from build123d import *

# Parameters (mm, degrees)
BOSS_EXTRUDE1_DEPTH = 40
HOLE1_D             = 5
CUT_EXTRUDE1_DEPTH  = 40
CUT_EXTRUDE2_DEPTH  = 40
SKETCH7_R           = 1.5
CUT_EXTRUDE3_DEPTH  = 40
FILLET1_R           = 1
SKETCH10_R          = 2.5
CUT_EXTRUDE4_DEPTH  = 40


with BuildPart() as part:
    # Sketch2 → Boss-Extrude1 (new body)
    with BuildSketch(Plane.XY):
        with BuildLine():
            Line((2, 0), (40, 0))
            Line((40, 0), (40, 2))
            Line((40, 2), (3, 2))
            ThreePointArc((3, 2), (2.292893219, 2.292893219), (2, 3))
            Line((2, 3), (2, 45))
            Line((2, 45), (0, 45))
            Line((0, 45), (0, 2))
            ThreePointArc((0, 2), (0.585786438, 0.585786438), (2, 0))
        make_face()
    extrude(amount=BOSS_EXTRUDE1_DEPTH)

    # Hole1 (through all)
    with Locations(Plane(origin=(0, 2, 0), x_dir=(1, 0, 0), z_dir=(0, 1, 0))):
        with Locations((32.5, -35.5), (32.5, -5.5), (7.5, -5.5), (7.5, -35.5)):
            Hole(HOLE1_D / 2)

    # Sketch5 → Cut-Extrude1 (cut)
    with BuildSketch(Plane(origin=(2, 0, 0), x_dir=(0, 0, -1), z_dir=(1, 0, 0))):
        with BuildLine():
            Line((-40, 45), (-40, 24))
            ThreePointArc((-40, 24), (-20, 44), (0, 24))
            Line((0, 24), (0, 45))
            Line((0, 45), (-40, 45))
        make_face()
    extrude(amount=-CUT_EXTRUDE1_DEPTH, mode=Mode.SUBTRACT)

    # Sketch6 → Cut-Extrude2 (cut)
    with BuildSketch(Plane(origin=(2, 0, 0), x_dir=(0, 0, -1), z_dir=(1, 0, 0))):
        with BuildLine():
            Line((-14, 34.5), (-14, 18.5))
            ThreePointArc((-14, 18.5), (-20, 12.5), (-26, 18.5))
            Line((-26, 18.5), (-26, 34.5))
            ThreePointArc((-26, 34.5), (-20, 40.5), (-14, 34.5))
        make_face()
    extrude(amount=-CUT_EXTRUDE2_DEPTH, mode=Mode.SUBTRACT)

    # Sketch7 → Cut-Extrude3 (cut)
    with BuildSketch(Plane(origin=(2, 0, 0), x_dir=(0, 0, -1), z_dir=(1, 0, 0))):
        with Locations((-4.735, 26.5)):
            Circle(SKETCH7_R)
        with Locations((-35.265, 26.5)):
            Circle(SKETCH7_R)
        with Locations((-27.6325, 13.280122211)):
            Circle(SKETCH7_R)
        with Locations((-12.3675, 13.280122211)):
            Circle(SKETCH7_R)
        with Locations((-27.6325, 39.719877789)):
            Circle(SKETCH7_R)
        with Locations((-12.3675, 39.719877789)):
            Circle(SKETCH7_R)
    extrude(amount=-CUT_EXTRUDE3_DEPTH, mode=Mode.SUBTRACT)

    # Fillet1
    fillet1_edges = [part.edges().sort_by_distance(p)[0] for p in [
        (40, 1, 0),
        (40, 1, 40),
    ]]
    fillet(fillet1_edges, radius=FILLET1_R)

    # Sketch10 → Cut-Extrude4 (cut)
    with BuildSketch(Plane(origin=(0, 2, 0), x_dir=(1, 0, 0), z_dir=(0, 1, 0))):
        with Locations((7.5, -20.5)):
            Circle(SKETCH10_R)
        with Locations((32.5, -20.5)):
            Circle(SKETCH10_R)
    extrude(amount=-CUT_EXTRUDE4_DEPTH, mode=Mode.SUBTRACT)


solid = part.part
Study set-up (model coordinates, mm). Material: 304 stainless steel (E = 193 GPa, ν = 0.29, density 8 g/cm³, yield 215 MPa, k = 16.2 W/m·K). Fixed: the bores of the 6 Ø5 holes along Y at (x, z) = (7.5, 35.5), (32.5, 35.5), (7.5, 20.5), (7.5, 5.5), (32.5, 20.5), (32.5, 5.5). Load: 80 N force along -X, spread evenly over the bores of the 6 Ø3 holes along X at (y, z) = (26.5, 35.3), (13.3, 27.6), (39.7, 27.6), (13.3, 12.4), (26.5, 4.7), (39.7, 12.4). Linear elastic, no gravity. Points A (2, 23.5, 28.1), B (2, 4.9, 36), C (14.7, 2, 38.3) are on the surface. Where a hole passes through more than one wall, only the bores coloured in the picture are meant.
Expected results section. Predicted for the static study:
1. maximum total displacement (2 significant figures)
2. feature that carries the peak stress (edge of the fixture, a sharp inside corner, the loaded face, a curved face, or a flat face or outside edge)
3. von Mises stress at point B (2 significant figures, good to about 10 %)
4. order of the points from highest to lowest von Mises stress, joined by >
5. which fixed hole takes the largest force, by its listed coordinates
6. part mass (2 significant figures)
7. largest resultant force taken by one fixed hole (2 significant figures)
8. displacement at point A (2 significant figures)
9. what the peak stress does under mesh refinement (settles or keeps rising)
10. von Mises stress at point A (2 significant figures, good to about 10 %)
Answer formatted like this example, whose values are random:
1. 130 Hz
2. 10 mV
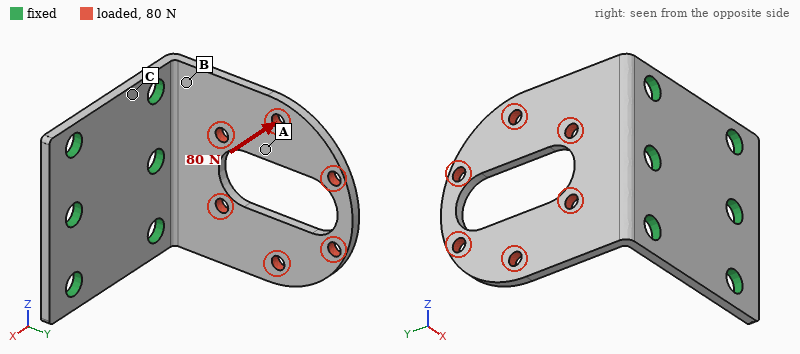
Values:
1. 0.28 mm
2. edge of the fixture
3. 61 MPa
4. B > A > C
5. (7.5, 20.5)
6. 42 g
7. 41 N
8. 0.11 mm
9. keeps rising
10. 33 MPa
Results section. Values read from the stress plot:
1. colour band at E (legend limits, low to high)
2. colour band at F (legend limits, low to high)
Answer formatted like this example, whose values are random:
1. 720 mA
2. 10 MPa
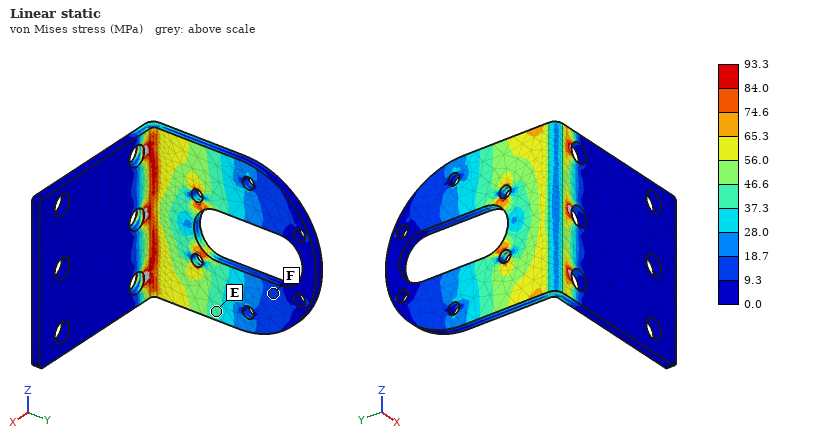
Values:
1. 37.3 to 46.6 MPa
2. 9.3 to 18.7 MPa
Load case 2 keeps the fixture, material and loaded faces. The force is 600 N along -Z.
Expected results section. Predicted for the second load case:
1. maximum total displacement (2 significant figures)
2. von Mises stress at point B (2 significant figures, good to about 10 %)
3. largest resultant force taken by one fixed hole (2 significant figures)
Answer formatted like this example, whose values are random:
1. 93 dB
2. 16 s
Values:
1. 51 µm
2. 68 MPa
3. 530 N
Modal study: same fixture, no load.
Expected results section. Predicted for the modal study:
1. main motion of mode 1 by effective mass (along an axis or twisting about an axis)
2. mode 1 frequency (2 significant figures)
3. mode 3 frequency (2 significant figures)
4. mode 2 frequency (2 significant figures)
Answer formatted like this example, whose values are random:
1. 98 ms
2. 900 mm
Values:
1. along X
2. 1000 Hz
3. 4900 Hz
4. 2300 Hz
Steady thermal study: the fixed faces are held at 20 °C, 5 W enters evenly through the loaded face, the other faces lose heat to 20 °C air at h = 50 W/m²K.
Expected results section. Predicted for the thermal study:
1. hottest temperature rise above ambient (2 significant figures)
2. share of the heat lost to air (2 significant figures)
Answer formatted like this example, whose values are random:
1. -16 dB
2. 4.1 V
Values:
1. 54 K
2. 73 %
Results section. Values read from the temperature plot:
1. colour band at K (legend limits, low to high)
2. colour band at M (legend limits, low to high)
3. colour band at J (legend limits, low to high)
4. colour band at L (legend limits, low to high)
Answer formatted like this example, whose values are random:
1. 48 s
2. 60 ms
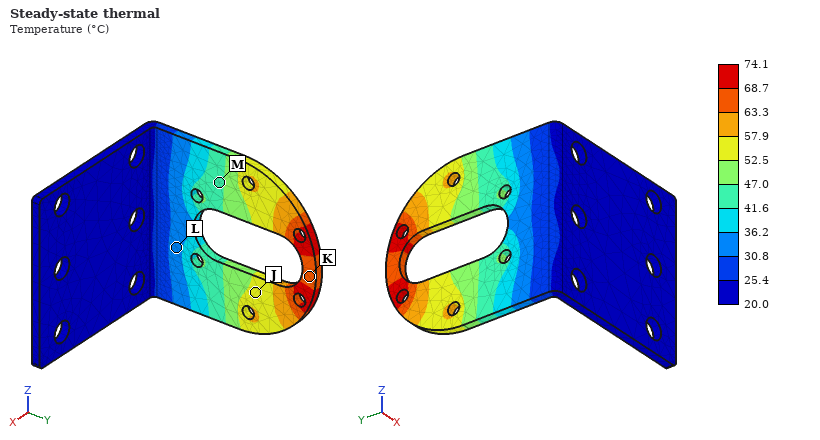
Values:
1. 63.3 to 68.7 °C
2. 41.6 to 47.0 °C
3. 52.5 to 57.9 °C
4. 30.8 to 36.2 °C
